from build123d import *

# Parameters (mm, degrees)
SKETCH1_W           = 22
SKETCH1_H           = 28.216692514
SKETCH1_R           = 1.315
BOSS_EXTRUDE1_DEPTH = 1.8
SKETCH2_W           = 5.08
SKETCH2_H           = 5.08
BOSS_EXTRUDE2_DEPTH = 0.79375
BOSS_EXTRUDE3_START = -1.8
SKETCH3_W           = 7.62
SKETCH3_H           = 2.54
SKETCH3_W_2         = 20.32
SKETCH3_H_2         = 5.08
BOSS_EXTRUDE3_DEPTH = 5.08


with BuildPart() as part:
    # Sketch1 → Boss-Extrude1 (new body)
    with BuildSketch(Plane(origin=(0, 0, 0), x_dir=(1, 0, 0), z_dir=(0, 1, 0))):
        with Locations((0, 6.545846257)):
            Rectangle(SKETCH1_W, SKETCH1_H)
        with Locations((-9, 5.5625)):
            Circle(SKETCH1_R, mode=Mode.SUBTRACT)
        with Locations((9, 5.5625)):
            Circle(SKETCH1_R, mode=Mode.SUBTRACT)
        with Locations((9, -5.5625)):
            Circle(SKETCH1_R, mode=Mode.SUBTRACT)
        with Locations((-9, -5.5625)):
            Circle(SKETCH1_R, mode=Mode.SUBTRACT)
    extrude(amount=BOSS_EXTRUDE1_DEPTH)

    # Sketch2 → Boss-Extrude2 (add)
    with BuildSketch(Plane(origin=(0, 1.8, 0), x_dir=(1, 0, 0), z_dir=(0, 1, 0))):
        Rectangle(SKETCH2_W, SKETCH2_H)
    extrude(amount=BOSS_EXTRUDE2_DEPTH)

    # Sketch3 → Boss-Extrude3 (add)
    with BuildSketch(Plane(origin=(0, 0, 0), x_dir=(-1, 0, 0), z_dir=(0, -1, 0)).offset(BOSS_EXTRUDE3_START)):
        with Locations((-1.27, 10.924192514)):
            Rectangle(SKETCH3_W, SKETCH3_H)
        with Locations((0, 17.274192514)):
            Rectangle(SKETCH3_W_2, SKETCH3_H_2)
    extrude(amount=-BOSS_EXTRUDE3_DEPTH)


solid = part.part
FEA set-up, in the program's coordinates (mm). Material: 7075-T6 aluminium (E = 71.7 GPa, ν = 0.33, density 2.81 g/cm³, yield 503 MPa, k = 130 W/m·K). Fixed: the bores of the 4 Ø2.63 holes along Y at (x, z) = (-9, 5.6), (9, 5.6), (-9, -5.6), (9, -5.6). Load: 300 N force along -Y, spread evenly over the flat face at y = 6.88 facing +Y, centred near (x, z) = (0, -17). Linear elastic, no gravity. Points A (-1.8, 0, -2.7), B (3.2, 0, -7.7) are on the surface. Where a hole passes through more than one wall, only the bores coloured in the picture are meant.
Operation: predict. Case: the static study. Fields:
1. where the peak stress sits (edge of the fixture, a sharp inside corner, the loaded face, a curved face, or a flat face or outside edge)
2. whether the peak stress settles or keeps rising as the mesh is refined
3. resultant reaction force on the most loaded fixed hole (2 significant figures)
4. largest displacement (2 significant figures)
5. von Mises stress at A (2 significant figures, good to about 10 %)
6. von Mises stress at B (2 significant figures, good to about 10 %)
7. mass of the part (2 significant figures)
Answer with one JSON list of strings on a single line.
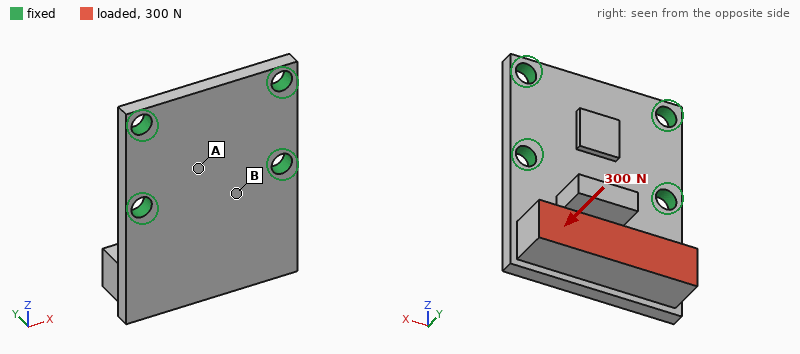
["edge of the fixture", "keeps rising", "190 N", "0.30 mm", "60 MPa", "150 MPa", "4.8 g"]
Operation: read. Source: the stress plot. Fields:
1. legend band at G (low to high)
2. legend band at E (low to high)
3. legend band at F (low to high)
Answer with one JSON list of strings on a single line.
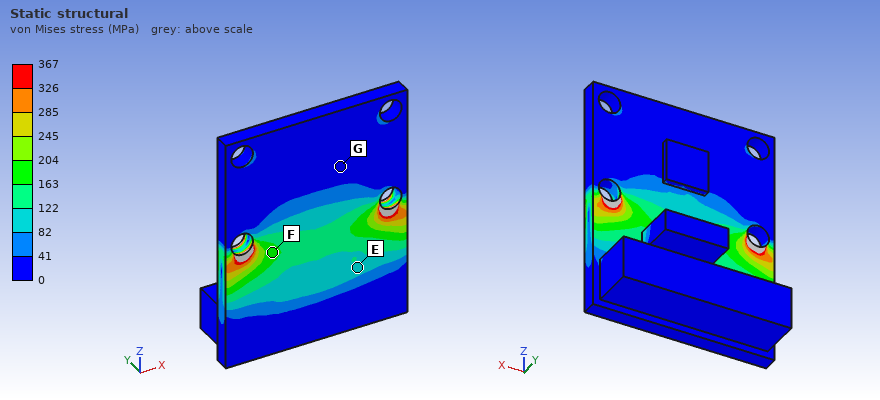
["0 to 41 MPa", "82 to 122 MPa", "163 to 204 MPa"]
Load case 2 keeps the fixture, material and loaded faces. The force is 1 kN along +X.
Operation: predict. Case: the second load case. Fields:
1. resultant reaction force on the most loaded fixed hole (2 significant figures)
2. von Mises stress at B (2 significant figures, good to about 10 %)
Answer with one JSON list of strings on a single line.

["850 N", "63 MPa"]
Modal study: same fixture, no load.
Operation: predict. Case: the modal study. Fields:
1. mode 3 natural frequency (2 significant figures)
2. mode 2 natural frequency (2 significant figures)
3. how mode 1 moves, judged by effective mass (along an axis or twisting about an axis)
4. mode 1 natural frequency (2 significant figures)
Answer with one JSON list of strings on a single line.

["19 kHz", "11 kHz", "along Y", "3700 Hz"]
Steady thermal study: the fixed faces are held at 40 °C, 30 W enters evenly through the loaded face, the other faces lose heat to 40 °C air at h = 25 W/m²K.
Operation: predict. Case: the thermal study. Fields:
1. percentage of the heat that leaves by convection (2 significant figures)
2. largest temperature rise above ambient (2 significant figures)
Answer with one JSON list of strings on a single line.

["4.3 %", "76 K"]
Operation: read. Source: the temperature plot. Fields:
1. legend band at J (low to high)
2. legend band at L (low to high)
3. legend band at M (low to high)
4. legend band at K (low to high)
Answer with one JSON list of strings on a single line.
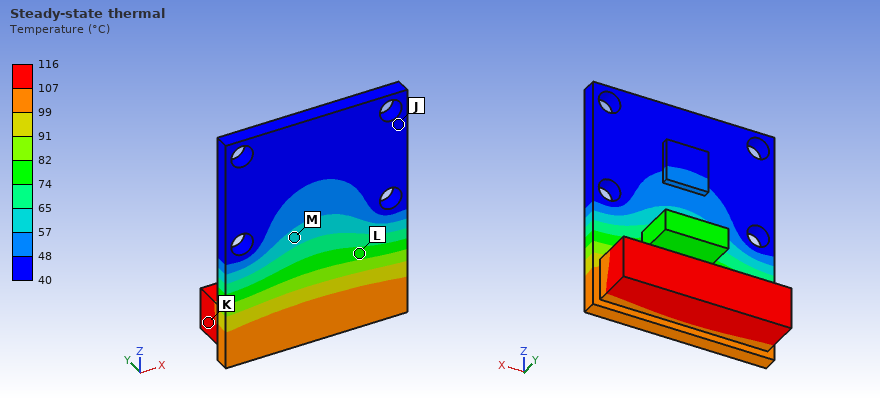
["40 to 48 °C", "74 to 82 °C", "57 to 65 °C", "107 to 116 °C"]
